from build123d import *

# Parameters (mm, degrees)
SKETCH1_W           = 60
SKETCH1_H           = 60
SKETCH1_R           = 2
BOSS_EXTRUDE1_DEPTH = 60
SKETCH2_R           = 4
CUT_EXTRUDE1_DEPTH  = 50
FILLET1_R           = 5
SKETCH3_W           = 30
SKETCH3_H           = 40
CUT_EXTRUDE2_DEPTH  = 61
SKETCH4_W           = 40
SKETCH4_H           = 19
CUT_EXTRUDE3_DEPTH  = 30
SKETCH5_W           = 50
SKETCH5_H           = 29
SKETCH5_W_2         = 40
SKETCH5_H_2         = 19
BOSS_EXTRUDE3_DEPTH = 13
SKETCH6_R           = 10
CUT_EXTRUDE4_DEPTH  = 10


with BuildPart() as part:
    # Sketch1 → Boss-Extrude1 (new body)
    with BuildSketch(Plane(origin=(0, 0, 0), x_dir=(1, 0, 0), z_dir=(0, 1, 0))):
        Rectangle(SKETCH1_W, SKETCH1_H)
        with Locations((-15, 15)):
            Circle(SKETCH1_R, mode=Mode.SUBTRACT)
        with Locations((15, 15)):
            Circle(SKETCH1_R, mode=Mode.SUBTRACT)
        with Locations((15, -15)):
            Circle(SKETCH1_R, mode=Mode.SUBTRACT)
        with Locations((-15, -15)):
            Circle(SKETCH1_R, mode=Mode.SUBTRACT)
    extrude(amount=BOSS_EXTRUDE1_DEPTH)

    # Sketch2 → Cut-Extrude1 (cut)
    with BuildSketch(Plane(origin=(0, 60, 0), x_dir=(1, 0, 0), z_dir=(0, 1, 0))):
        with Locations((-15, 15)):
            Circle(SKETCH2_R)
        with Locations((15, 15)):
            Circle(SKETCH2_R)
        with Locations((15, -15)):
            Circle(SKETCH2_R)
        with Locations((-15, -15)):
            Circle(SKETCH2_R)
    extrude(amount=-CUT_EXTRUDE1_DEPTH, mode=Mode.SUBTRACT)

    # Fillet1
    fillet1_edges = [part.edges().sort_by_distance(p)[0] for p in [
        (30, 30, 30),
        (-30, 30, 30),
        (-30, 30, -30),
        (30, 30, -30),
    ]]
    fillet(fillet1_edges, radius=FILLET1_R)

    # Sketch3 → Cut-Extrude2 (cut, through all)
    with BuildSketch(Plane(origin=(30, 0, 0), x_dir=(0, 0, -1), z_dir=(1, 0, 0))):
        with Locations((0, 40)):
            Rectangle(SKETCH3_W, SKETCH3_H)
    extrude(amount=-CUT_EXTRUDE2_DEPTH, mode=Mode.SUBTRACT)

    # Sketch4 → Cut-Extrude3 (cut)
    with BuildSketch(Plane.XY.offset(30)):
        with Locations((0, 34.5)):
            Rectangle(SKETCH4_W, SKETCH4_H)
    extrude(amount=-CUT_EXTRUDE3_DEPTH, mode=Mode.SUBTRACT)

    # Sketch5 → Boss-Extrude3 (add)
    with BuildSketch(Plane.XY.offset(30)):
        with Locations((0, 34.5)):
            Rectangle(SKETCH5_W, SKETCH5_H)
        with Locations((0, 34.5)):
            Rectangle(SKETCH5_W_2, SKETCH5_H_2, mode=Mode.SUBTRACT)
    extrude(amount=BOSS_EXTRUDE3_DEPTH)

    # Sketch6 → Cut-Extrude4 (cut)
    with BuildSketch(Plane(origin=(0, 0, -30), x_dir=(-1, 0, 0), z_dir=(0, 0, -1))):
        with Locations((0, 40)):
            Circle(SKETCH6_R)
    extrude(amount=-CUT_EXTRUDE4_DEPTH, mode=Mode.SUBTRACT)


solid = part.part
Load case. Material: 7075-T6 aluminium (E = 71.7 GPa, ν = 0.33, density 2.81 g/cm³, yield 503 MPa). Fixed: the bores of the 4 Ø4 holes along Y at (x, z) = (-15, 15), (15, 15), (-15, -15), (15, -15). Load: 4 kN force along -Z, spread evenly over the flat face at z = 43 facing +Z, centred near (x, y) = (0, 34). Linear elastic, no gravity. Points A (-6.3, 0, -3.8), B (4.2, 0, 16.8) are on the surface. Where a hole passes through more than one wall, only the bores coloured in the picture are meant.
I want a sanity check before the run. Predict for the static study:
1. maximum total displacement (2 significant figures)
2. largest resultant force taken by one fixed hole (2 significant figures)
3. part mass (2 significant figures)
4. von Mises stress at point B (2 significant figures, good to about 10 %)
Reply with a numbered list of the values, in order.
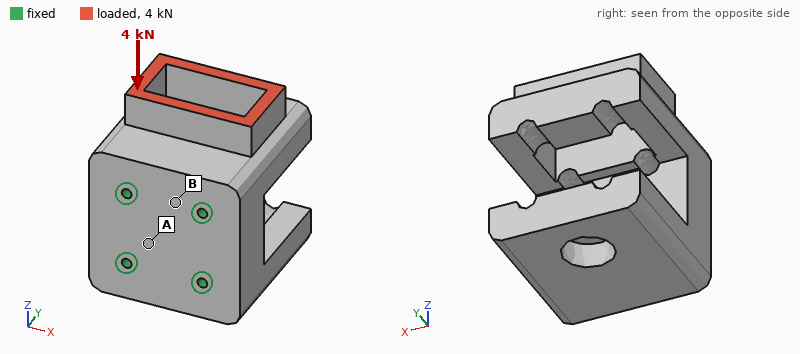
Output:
1. 0.10 mm
2. 2.3 kN
3. 370 g
4. 12 MPa
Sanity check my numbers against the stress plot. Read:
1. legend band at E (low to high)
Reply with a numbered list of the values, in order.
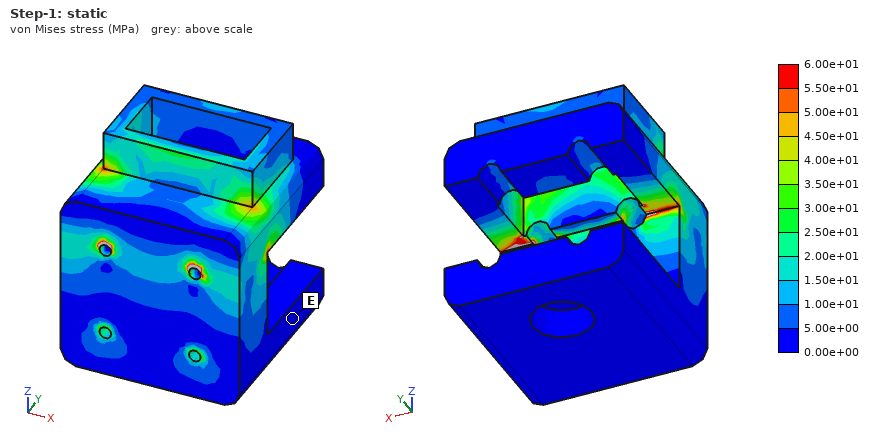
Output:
1. 0.00e+00 to 5.00e+00 MPa
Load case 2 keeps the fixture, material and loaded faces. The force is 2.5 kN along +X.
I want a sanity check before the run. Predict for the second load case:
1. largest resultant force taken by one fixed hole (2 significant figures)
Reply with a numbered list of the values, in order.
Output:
1. 2.3 kN
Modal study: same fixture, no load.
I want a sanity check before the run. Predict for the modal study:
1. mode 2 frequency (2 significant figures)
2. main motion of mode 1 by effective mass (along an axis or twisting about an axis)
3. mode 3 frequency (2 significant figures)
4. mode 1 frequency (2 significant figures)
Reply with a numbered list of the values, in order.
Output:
1. 4100 Hz
2. along Z
3. 4200 Hz
4. 3200 Hz
